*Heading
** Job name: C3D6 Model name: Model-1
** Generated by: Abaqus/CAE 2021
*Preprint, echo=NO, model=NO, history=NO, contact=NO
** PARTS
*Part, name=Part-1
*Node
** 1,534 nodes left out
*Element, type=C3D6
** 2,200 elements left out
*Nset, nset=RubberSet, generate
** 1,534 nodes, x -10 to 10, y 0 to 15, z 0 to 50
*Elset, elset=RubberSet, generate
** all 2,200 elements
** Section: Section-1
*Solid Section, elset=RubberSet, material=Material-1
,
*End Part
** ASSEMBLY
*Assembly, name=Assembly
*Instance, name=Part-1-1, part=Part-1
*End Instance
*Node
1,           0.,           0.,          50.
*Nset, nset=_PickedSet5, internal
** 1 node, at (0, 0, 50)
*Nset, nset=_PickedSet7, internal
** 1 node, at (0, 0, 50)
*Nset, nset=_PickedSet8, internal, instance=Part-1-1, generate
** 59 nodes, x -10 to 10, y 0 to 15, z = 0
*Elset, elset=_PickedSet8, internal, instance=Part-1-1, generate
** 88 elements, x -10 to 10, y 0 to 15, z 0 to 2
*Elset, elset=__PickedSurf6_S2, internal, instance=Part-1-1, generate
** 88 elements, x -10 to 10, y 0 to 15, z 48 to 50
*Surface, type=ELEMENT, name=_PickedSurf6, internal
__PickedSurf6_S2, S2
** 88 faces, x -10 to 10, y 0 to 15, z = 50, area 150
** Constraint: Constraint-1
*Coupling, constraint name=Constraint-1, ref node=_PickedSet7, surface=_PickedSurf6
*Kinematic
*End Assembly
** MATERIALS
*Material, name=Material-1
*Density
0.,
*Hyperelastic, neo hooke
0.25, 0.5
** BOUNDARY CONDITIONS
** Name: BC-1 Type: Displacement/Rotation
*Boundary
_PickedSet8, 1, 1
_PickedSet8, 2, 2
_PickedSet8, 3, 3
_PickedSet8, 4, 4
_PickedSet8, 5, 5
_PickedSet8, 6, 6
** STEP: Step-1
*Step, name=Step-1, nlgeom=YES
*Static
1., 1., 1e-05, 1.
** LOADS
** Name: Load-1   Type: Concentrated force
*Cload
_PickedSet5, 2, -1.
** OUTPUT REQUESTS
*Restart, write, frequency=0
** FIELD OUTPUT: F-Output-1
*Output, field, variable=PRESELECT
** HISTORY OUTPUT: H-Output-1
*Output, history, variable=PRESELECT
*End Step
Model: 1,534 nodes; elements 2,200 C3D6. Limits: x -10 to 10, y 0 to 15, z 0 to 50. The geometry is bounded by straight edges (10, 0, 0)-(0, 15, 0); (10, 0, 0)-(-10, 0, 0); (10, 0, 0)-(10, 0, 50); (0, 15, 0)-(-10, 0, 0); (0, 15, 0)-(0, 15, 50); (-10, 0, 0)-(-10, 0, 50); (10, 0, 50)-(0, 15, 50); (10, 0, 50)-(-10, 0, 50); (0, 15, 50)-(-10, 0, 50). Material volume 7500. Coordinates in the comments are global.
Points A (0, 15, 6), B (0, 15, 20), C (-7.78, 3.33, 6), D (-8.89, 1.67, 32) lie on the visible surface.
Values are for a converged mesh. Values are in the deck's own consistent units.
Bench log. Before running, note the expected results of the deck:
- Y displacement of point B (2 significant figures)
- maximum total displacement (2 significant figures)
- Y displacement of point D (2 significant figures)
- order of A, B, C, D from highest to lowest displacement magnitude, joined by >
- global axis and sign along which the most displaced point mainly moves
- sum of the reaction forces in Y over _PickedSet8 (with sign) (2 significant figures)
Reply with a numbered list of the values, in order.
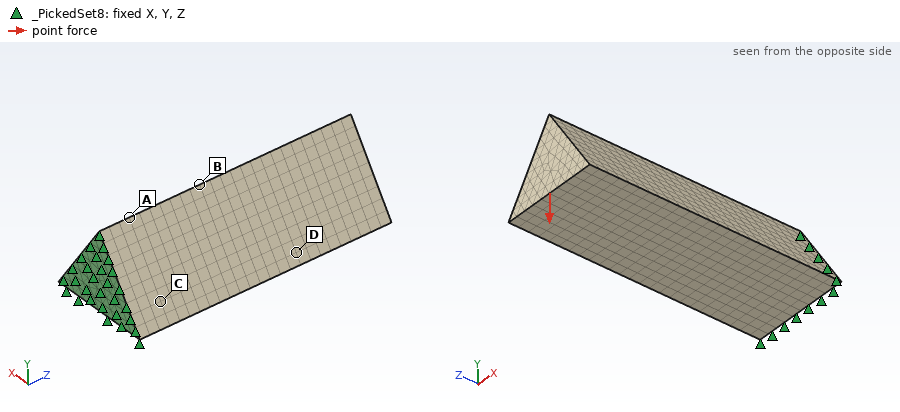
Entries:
1. -3.8
2. 15
3. -6.9
4. D > B > A > C
5. -Y
6. 1.0
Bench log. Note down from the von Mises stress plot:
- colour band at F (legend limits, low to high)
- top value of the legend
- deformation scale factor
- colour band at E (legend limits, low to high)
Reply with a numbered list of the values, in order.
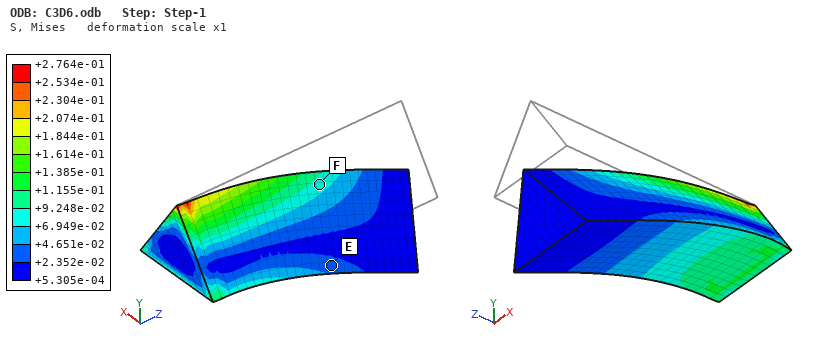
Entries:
1. +6.949e-02 to +9.248e-02
2. +2.764e-01
3. 1
4. +2.352e-02 to +4.651e-02
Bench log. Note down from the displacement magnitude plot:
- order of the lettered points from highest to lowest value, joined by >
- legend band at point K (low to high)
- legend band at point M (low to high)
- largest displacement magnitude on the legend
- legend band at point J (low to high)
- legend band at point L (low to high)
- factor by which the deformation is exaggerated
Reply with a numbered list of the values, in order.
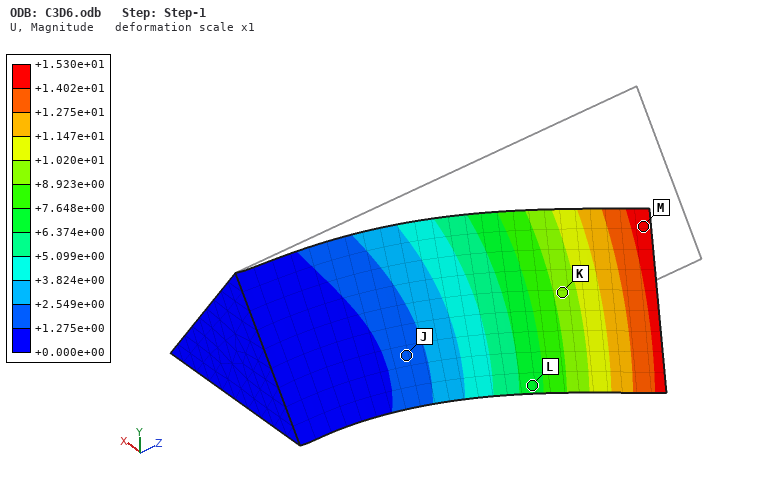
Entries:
1. M > K > L > J
2. +8.923e+00 to +1.020e+01
3. +1.402e+01 to +1.530e+01
4. +1.530e+01
5. +1.275e+00 to +2.549e+00
6. +6.374e+00 to +7.648e+00
7. 1
